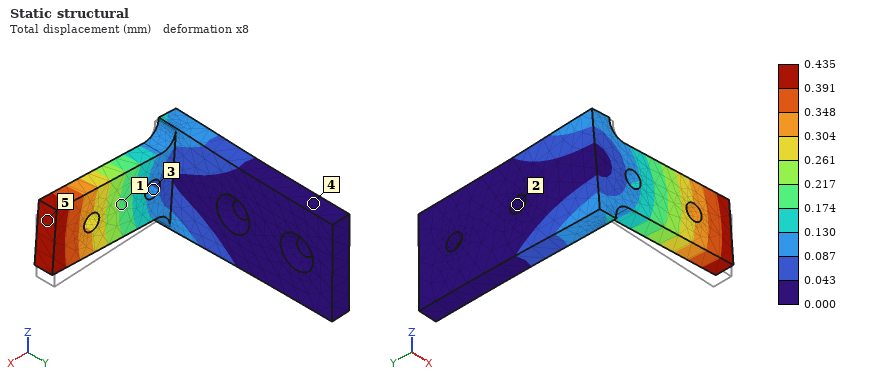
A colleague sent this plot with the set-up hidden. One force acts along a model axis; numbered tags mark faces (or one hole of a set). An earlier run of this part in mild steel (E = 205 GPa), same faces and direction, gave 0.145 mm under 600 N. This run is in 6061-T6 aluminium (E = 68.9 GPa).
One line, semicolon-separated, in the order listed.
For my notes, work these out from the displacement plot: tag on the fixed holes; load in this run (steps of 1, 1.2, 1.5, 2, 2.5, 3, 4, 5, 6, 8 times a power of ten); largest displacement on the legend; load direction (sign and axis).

2; 600 N; 0.435 mm; +Z
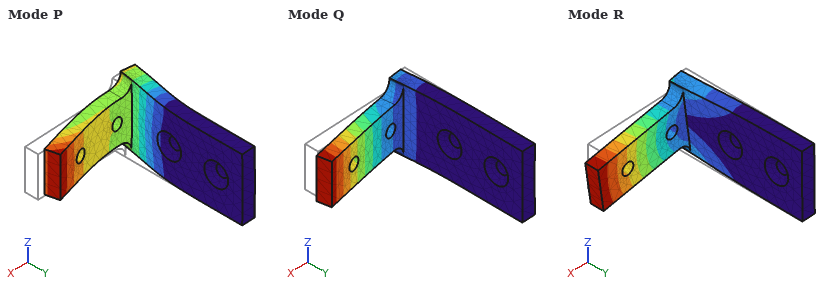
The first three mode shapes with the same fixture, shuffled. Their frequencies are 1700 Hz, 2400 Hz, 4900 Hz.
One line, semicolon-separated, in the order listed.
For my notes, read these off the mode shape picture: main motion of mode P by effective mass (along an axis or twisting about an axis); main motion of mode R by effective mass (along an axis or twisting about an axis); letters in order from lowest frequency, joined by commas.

along X; along Z; Q, R, P
